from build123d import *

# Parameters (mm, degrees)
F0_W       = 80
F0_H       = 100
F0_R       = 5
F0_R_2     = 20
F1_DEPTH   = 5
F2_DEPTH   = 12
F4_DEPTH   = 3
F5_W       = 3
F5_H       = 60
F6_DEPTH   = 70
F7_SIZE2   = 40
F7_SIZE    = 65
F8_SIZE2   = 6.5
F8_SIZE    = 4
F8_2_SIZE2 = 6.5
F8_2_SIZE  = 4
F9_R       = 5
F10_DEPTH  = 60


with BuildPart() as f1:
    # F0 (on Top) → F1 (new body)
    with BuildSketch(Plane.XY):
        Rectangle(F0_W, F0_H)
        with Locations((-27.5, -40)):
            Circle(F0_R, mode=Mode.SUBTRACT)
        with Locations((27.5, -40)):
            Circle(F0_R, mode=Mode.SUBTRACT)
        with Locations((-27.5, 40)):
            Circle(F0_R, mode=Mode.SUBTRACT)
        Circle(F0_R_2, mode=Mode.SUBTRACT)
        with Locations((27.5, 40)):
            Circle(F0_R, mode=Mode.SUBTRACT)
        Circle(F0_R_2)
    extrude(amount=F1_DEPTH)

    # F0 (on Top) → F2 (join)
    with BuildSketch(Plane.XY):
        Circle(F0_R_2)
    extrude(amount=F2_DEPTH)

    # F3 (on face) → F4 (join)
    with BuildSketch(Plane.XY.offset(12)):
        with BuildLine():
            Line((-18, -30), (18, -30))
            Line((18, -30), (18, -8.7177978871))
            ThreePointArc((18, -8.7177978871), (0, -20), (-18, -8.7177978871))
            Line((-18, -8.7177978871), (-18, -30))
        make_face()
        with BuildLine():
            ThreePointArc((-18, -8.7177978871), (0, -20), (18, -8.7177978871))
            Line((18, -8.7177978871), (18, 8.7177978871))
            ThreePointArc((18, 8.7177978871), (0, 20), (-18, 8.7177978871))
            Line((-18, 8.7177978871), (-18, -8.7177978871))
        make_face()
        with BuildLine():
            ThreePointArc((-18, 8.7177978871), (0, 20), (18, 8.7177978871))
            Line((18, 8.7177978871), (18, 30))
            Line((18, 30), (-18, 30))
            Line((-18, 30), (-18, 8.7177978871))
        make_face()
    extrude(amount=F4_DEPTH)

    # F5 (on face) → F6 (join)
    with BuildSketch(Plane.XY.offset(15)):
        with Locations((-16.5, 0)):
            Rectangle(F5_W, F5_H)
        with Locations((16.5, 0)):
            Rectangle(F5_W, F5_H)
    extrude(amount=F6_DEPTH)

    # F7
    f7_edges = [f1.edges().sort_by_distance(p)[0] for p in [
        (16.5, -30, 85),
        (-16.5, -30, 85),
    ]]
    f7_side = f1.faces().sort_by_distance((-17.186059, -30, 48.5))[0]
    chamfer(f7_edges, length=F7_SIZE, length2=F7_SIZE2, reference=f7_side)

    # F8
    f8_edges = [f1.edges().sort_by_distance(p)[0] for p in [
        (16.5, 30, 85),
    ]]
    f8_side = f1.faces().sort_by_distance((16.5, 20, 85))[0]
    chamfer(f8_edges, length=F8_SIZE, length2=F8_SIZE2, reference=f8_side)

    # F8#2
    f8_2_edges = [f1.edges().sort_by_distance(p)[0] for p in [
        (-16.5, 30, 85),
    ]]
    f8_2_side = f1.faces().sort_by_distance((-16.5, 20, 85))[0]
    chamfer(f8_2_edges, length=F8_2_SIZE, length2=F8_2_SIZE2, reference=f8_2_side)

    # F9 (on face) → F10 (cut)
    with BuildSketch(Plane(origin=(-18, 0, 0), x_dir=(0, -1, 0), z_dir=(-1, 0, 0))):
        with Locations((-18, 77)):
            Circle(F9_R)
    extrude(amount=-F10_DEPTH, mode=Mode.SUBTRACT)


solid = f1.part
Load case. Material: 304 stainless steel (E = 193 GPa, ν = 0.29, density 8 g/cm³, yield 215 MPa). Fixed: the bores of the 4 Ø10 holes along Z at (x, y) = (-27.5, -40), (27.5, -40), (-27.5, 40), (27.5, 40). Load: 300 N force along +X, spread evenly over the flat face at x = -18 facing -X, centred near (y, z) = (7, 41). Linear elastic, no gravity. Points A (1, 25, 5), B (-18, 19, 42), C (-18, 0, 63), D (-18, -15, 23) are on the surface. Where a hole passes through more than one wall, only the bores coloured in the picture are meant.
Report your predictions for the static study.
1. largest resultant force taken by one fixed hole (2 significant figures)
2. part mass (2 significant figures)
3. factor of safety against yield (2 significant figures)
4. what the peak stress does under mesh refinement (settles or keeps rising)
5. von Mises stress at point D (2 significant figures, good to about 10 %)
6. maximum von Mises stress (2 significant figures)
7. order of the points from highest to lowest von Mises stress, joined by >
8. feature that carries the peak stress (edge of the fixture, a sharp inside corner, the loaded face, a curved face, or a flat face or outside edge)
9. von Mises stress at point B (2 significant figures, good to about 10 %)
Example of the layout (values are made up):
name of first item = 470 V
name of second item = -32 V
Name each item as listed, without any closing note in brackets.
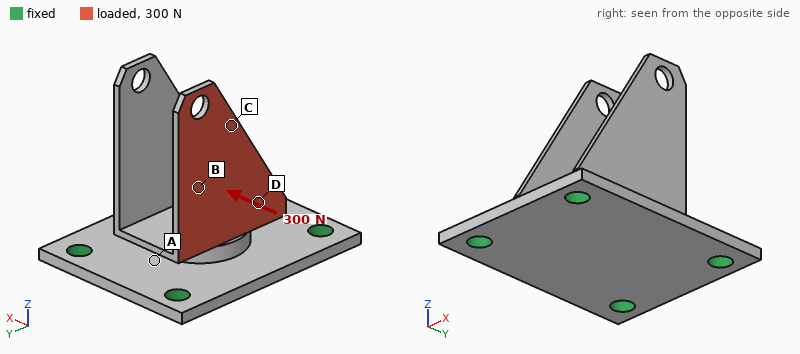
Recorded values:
largest resultant force taken by one fixed hole = 160 N
part mass = 560 g
factor of safety against yield = 2.0
what the peak stress does under mesh refinement = settles
von Mises stress at point D = 54 MPa
maximum von Mises stress = 110 MPa
order of the points from highest to lowest von Mises stress, joined by > = D > B > C > A
feature that carries the peak stress = the loaded face
von Mises stress at point B = 34 MPa
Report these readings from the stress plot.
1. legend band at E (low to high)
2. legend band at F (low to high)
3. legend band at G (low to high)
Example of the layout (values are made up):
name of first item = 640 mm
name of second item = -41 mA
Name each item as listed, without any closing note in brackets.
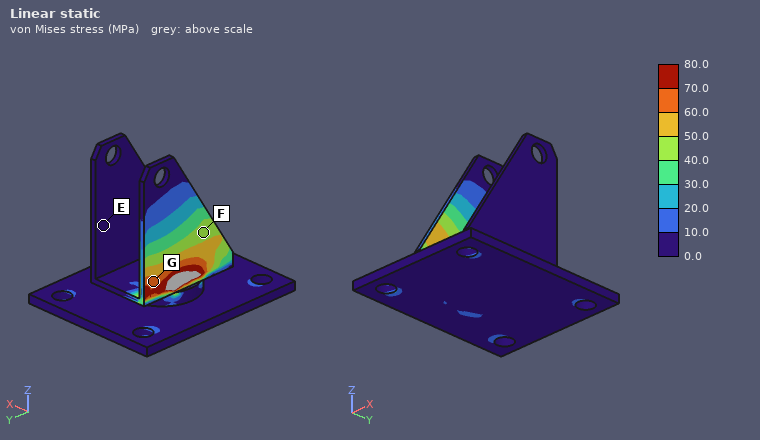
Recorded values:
legend band at E = 0.0 to 10.0 MPa
legend band at F = 40.0 to 50.0 MPa
legend band at G = 60.0 to 70.0 MPa
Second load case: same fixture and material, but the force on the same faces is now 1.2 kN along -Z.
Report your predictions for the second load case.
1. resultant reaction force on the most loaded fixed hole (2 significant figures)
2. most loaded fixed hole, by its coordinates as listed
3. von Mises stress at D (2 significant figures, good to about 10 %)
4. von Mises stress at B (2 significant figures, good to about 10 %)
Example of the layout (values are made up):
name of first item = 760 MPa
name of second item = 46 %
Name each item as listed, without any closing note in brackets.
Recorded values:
resultant reaction force on the most loaded fixed hole = 600 N
most loaded fixed hole, by its coordinates as listed = (-27.5, 40)
von Mises stress at D = 16 MPa
von Mises stress at B = 17 MPa
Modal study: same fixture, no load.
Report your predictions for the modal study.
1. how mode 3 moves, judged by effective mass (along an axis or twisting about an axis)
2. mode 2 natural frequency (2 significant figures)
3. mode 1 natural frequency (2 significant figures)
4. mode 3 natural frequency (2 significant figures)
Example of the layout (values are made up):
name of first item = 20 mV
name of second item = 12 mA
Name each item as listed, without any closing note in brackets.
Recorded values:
how mode 3 moves, judged by effective mass = along Y
mode 2 natural frequency = 640 Hz
mode 1 natural frequency = 620 Hz
mode 3 natural frequency = 2200 Hz
